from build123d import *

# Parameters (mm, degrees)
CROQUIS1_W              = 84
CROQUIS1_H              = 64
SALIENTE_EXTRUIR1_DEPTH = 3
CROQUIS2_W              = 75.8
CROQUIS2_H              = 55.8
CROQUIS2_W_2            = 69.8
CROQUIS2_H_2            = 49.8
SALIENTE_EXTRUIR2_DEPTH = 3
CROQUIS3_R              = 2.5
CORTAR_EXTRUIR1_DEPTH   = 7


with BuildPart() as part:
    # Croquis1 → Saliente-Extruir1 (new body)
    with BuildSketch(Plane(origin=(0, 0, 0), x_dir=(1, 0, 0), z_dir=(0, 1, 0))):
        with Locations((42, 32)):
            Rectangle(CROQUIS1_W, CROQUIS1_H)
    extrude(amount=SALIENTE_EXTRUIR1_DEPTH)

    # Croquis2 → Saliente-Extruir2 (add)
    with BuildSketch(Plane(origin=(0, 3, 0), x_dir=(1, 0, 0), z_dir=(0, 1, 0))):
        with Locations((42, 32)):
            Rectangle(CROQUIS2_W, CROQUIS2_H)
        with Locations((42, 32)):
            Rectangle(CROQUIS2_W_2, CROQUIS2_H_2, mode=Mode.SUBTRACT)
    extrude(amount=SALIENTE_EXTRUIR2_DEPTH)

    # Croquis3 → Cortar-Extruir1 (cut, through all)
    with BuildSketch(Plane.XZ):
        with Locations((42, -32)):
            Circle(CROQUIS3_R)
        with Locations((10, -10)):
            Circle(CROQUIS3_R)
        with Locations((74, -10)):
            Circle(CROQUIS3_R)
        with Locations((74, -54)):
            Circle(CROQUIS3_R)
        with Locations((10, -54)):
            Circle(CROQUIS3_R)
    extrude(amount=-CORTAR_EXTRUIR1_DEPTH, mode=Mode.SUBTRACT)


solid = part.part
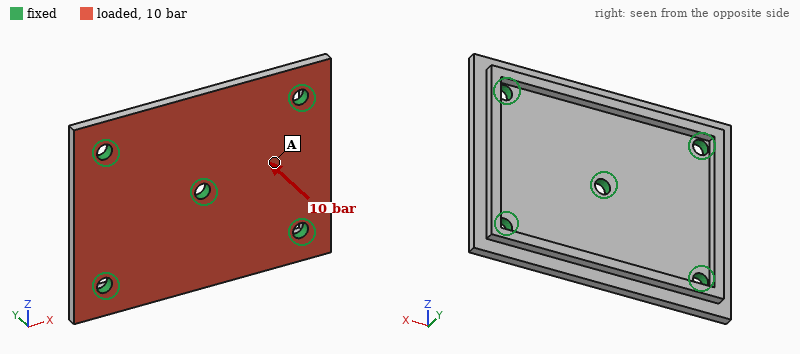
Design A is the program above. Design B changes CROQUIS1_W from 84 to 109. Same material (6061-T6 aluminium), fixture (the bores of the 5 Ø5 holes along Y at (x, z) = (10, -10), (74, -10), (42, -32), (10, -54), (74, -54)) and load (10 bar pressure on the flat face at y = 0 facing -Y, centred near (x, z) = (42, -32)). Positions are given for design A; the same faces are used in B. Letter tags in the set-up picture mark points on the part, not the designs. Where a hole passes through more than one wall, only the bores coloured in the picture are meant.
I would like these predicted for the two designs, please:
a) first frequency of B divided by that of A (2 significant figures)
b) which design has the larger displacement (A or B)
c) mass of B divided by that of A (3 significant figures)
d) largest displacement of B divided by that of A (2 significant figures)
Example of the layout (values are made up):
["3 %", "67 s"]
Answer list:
["0.77", "B", "1.27", "2.0"]
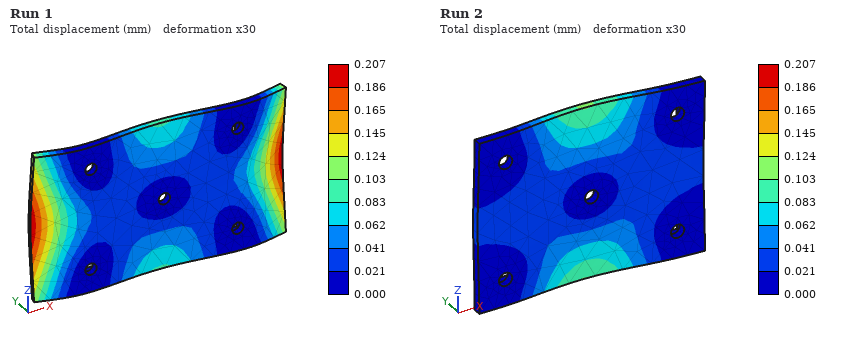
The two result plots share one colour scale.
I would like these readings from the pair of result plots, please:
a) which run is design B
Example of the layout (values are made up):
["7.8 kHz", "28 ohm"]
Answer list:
["Run 1"]
